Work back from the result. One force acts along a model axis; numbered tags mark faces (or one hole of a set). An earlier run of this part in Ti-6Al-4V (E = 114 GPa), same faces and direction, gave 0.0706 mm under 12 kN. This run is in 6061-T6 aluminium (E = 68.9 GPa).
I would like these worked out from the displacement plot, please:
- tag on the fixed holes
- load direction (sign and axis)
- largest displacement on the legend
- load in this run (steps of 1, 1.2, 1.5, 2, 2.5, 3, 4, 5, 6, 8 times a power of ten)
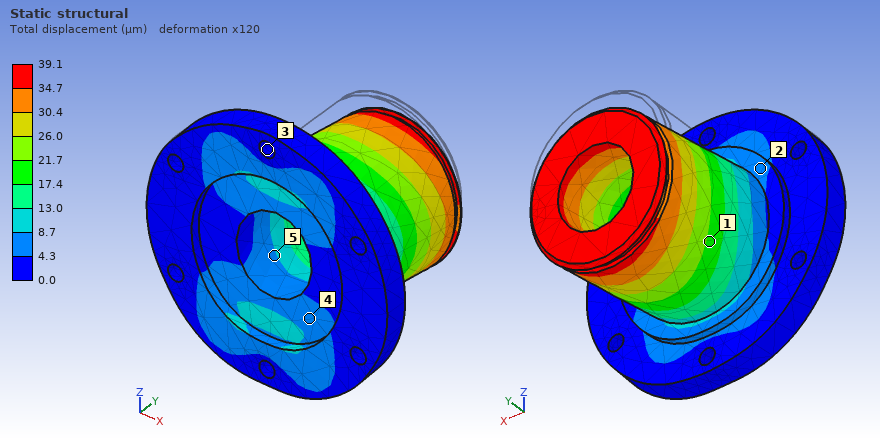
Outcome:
3
-Z
39.1 µm
4 kN
